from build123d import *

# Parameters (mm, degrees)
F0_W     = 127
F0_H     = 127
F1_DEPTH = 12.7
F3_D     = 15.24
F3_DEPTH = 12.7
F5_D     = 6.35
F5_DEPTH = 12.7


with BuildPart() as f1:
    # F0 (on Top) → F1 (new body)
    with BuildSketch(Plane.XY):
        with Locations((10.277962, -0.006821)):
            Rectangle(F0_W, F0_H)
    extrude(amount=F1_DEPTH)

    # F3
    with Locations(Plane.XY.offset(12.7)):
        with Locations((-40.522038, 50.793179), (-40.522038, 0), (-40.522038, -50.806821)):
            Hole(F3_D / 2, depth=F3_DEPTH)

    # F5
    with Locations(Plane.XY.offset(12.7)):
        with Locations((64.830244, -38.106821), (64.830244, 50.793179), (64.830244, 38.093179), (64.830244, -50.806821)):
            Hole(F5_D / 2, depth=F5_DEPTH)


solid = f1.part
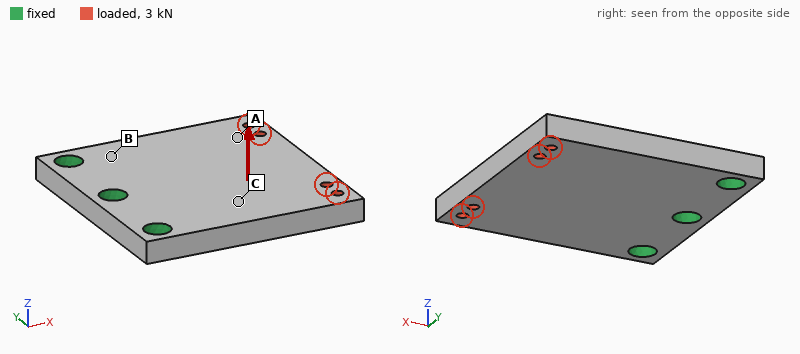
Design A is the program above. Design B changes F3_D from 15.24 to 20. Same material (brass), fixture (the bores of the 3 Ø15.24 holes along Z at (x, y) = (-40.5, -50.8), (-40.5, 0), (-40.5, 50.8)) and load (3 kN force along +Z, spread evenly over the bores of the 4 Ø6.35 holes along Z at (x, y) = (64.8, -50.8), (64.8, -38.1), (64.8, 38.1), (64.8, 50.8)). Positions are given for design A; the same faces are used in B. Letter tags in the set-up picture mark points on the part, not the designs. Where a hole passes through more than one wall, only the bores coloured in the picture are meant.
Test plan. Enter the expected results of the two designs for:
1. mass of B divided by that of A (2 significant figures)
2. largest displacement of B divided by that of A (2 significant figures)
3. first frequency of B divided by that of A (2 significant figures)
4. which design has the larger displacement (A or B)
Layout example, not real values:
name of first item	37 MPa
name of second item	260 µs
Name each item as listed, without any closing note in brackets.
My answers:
mass of B divided by that of A	0.97
largest displacement of B divided by that of A	0.91
first frequency of B divided by that of A	1.1
which design has the larger displacement	A
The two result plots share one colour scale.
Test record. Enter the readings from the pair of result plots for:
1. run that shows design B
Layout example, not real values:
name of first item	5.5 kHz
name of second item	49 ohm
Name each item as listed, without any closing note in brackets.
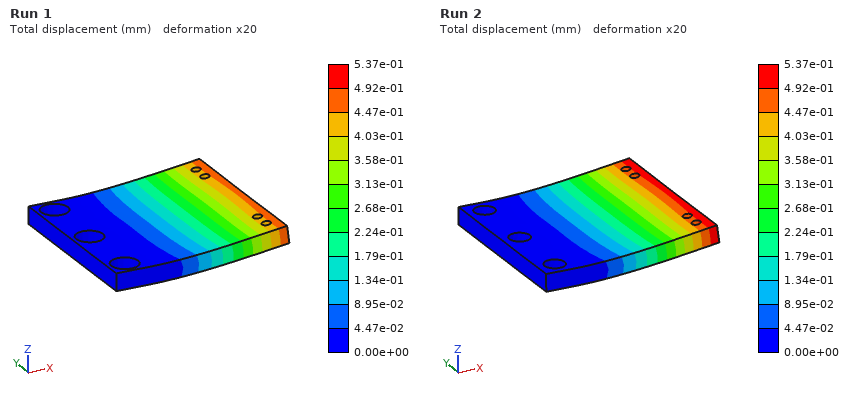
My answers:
run that shows design B	Run 1
